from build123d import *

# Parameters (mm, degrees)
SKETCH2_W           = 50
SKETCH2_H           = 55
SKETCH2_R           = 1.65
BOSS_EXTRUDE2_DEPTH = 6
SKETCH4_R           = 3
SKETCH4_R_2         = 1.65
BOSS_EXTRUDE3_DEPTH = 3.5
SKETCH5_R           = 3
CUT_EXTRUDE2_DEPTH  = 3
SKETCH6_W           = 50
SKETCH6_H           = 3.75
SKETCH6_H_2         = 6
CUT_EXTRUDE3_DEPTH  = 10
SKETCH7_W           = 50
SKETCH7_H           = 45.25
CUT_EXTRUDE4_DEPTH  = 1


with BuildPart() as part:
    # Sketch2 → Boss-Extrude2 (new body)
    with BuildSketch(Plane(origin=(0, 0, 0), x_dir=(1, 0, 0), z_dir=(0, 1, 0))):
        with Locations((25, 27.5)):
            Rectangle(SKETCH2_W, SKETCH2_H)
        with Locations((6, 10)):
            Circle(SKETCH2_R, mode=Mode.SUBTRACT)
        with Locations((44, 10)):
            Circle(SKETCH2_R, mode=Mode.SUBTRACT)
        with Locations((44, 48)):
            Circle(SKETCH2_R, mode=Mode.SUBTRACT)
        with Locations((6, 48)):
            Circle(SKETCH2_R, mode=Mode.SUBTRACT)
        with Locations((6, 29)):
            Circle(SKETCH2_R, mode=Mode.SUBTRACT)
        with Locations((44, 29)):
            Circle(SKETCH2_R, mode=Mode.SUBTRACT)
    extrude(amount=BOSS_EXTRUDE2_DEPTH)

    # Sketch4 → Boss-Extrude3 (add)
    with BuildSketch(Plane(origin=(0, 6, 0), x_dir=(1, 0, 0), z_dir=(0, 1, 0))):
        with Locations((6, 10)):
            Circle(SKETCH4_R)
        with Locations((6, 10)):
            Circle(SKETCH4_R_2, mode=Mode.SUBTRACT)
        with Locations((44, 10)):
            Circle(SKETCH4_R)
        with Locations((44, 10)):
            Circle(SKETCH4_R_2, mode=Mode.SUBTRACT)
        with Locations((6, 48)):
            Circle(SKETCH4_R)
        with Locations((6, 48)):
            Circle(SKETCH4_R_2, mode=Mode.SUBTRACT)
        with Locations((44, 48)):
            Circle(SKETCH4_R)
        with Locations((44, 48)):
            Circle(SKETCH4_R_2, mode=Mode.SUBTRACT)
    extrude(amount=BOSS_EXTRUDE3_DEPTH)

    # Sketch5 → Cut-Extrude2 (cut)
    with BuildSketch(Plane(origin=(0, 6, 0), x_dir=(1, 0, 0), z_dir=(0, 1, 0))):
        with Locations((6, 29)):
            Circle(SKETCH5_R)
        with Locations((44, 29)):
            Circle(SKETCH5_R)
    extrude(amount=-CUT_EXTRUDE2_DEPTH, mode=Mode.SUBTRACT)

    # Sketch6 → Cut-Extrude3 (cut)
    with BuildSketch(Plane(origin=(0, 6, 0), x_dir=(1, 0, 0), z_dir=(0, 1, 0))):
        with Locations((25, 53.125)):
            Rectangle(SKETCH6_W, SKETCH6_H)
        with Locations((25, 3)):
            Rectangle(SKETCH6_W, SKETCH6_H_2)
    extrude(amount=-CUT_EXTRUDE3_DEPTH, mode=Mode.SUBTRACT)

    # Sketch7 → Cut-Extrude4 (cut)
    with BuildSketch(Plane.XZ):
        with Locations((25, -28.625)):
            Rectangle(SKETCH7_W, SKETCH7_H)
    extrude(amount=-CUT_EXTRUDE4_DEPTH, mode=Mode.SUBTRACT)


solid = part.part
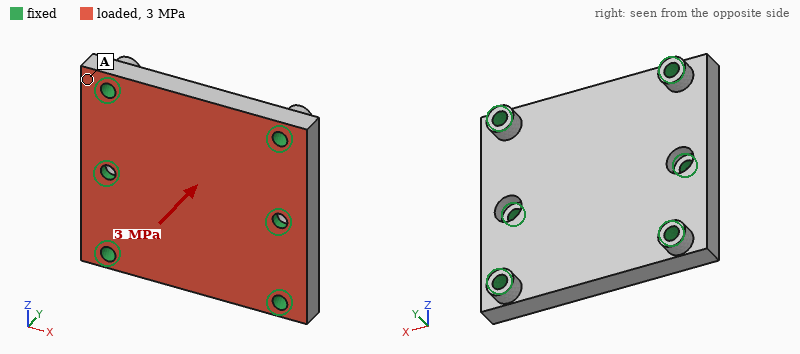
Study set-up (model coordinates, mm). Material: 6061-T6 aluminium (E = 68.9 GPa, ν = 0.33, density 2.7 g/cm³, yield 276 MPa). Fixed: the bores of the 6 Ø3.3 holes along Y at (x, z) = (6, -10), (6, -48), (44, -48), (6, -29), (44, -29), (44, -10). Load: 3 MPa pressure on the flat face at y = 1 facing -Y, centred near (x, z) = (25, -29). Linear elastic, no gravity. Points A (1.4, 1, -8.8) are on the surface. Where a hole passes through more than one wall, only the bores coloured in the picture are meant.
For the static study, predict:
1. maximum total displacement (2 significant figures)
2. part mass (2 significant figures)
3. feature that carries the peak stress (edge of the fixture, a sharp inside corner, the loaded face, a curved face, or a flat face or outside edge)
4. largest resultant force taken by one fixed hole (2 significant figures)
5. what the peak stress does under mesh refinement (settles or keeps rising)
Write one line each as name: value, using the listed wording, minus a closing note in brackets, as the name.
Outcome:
maximum total displacement: 36 µm
part mass: 30 g
feature that carries the peak stress: edge of the fixture
largest resultant force taken by one fixed hole: 1.3 kN
what the peak stress does under mesh refinement: keeps rising
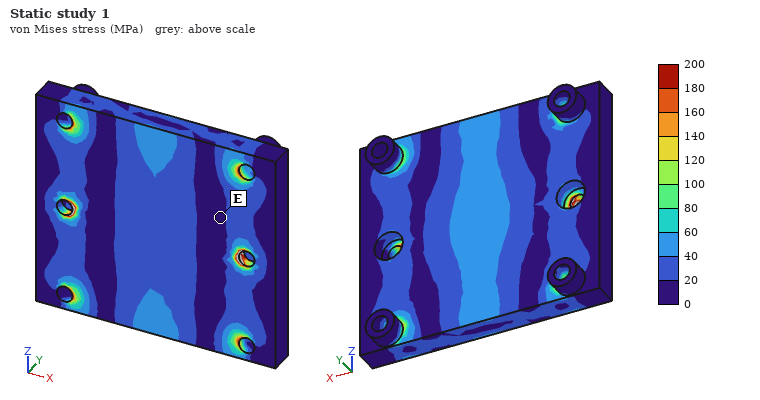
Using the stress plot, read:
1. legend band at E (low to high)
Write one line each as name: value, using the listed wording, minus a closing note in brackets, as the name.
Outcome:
legend band at E: 0 to 20 MPa
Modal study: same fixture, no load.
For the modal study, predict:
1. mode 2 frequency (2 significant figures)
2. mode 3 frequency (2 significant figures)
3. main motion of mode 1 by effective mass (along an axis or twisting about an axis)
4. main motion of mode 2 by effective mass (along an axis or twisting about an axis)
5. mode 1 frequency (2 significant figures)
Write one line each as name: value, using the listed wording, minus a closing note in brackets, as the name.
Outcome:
mode 2 frequency: 19 kHz
mode 3 frequency: 26 kHz
main motion of mode 1 by effective mass: along Y
main motion of mode 2 by effective mass: twisting about X
mode 1 frequency: 14 kHz
